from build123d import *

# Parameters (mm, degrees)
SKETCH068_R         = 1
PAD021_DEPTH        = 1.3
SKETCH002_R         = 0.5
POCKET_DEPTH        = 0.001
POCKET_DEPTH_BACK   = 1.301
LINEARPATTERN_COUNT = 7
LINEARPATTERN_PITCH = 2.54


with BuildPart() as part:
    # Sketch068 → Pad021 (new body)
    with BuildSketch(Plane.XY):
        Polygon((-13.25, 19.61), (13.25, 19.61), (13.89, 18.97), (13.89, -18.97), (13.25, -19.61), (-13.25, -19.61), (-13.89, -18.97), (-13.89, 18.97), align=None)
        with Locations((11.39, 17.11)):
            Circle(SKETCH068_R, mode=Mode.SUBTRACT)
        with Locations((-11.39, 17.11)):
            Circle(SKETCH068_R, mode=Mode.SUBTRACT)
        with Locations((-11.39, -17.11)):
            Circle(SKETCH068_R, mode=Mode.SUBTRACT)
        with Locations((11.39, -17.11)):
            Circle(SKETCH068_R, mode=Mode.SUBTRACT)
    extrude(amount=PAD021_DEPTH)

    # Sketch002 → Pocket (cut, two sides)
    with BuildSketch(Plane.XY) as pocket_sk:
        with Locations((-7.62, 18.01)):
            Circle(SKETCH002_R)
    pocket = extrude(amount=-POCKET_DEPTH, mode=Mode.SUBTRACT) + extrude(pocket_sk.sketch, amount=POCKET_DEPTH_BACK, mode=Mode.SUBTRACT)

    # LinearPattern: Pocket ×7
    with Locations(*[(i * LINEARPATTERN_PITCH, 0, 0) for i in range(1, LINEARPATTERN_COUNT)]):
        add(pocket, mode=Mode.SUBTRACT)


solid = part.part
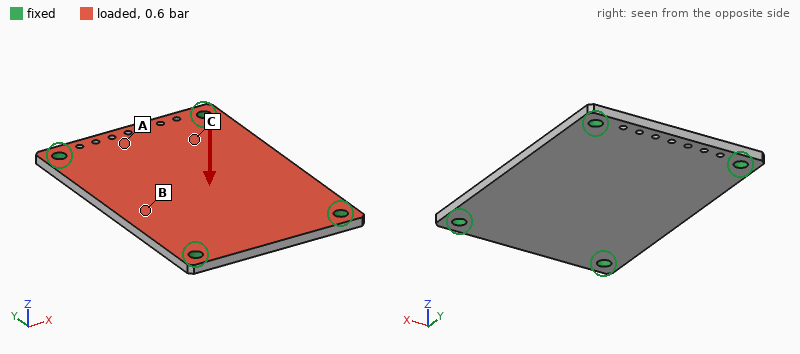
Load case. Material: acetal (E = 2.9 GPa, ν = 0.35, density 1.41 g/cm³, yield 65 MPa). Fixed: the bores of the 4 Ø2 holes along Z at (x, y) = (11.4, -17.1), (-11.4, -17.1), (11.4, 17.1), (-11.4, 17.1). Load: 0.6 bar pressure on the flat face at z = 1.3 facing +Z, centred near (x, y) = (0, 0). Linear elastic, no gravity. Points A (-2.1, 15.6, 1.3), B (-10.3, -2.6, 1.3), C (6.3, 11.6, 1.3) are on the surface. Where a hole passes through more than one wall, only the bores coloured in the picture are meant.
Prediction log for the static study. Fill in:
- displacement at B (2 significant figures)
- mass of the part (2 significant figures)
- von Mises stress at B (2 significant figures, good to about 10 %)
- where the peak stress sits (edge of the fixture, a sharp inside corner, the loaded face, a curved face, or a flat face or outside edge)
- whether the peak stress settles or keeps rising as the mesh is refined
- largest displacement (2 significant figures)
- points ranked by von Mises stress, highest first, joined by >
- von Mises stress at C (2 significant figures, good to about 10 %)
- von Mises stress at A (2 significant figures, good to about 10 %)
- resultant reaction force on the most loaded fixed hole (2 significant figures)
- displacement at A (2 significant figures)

0.48 mm
2.0 g
11 MPa
edge of the fixture
keeps rising
0.55 mm
B > A > C
3.5 MPa
6.1 MPa
16 N
0.14 mm
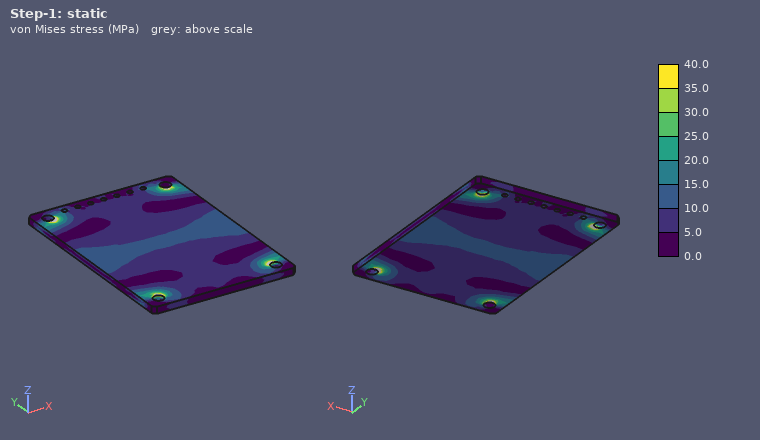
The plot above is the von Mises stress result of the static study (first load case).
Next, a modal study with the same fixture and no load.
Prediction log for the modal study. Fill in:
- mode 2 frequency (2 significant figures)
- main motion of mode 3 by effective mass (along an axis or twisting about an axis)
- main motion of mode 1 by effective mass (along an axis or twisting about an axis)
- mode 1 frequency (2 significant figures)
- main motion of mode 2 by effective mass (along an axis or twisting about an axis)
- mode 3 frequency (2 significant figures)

2200 Hz
twisting about X
along Z
1400 Hz
twisting about Y
3400 Hz
